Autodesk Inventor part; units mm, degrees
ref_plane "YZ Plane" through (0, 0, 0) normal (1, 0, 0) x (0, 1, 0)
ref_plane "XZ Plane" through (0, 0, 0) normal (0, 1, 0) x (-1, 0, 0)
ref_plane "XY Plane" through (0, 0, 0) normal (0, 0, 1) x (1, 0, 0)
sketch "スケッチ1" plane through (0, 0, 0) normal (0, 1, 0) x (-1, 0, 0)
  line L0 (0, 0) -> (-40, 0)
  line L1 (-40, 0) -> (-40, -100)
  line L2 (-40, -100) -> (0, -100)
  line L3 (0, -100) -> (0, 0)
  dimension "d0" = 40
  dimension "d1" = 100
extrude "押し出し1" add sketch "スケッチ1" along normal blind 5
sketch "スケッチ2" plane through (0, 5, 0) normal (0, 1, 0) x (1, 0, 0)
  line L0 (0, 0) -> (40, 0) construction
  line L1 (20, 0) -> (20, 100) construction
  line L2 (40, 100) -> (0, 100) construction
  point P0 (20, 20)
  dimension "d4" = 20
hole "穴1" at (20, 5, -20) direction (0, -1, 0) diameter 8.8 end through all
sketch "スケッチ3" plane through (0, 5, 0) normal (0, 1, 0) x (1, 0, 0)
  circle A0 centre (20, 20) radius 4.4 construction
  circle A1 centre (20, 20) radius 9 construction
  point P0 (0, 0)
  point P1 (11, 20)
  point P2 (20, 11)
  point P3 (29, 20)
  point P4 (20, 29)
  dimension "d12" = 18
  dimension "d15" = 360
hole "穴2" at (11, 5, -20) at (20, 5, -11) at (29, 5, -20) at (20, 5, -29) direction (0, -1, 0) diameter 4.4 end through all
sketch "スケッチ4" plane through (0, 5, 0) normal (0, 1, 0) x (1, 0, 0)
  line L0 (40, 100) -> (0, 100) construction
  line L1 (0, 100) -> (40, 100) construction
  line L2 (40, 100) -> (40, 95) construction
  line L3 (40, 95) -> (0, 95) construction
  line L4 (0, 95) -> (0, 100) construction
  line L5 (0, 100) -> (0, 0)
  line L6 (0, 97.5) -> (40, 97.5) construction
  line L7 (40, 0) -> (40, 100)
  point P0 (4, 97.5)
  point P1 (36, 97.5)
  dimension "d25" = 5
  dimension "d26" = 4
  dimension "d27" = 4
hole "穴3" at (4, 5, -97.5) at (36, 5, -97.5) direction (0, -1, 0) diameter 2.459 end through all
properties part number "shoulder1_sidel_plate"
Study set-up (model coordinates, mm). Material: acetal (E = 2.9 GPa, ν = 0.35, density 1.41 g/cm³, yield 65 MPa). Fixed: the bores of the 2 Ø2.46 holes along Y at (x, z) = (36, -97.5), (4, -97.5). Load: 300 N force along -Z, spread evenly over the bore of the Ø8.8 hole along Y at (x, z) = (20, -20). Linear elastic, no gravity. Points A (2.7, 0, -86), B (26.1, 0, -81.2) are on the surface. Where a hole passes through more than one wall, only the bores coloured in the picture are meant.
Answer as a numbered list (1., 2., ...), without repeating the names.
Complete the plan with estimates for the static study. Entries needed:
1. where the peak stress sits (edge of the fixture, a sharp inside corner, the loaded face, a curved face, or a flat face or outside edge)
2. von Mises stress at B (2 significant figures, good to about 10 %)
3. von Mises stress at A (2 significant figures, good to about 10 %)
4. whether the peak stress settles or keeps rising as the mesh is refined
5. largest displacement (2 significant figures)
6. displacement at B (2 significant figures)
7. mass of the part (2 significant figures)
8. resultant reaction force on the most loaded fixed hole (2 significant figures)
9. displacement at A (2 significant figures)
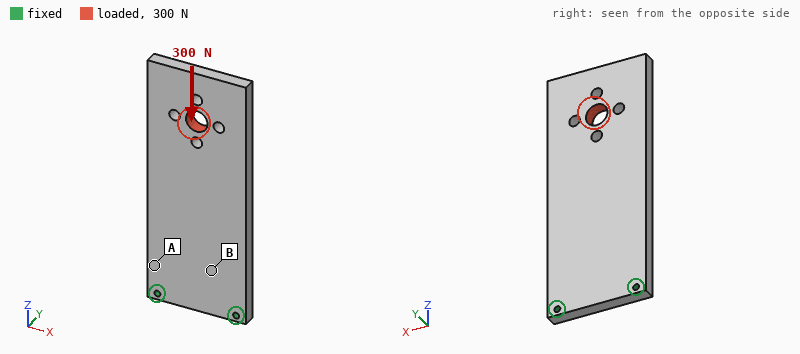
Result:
1. edge of the fixture
2. 1.2 MPa
3. 2.3 MPa
4. keeps rising
5. 63 µm
6. 17 µm
7. 27 g
8. 160 N
9. 12 µm
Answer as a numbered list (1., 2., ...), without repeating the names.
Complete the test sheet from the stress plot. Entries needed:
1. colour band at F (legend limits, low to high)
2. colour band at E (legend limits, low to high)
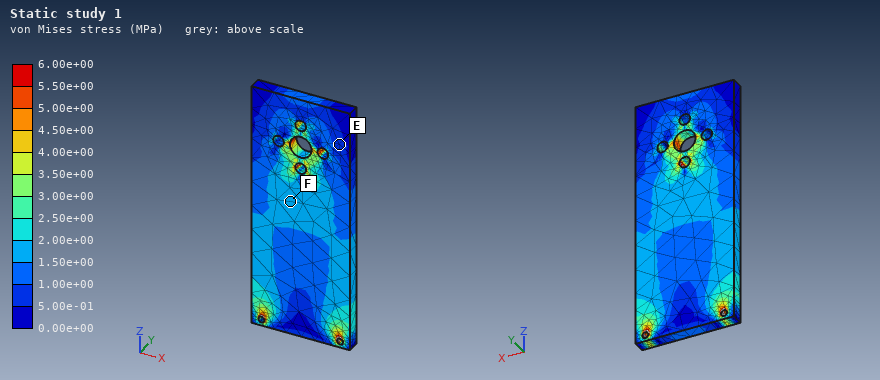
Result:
1. 1.50e+00 to 2.00e+00 MPa
2. 5.00e-01 to 1.00e+00 MPa
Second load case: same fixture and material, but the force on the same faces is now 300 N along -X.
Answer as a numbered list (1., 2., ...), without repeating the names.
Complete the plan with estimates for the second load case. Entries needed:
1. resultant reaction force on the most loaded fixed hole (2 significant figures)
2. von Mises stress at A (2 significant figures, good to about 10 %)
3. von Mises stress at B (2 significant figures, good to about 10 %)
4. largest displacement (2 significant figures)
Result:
1. 730 N
2. 13 MPa
3. 4.9 MPa
4. 1.1 mm
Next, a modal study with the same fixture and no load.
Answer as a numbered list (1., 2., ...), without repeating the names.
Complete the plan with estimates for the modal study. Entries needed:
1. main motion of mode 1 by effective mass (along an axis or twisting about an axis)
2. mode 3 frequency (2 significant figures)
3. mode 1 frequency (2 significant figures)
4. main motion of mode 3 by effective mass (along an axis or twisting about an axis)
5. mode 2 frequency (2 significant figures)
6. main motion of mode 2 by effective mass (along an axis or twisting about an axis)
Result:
1. along Y
2. 690 Hz
3. 110 Hz
4. along Y
5. 590 Hz
6. twisting about Z
